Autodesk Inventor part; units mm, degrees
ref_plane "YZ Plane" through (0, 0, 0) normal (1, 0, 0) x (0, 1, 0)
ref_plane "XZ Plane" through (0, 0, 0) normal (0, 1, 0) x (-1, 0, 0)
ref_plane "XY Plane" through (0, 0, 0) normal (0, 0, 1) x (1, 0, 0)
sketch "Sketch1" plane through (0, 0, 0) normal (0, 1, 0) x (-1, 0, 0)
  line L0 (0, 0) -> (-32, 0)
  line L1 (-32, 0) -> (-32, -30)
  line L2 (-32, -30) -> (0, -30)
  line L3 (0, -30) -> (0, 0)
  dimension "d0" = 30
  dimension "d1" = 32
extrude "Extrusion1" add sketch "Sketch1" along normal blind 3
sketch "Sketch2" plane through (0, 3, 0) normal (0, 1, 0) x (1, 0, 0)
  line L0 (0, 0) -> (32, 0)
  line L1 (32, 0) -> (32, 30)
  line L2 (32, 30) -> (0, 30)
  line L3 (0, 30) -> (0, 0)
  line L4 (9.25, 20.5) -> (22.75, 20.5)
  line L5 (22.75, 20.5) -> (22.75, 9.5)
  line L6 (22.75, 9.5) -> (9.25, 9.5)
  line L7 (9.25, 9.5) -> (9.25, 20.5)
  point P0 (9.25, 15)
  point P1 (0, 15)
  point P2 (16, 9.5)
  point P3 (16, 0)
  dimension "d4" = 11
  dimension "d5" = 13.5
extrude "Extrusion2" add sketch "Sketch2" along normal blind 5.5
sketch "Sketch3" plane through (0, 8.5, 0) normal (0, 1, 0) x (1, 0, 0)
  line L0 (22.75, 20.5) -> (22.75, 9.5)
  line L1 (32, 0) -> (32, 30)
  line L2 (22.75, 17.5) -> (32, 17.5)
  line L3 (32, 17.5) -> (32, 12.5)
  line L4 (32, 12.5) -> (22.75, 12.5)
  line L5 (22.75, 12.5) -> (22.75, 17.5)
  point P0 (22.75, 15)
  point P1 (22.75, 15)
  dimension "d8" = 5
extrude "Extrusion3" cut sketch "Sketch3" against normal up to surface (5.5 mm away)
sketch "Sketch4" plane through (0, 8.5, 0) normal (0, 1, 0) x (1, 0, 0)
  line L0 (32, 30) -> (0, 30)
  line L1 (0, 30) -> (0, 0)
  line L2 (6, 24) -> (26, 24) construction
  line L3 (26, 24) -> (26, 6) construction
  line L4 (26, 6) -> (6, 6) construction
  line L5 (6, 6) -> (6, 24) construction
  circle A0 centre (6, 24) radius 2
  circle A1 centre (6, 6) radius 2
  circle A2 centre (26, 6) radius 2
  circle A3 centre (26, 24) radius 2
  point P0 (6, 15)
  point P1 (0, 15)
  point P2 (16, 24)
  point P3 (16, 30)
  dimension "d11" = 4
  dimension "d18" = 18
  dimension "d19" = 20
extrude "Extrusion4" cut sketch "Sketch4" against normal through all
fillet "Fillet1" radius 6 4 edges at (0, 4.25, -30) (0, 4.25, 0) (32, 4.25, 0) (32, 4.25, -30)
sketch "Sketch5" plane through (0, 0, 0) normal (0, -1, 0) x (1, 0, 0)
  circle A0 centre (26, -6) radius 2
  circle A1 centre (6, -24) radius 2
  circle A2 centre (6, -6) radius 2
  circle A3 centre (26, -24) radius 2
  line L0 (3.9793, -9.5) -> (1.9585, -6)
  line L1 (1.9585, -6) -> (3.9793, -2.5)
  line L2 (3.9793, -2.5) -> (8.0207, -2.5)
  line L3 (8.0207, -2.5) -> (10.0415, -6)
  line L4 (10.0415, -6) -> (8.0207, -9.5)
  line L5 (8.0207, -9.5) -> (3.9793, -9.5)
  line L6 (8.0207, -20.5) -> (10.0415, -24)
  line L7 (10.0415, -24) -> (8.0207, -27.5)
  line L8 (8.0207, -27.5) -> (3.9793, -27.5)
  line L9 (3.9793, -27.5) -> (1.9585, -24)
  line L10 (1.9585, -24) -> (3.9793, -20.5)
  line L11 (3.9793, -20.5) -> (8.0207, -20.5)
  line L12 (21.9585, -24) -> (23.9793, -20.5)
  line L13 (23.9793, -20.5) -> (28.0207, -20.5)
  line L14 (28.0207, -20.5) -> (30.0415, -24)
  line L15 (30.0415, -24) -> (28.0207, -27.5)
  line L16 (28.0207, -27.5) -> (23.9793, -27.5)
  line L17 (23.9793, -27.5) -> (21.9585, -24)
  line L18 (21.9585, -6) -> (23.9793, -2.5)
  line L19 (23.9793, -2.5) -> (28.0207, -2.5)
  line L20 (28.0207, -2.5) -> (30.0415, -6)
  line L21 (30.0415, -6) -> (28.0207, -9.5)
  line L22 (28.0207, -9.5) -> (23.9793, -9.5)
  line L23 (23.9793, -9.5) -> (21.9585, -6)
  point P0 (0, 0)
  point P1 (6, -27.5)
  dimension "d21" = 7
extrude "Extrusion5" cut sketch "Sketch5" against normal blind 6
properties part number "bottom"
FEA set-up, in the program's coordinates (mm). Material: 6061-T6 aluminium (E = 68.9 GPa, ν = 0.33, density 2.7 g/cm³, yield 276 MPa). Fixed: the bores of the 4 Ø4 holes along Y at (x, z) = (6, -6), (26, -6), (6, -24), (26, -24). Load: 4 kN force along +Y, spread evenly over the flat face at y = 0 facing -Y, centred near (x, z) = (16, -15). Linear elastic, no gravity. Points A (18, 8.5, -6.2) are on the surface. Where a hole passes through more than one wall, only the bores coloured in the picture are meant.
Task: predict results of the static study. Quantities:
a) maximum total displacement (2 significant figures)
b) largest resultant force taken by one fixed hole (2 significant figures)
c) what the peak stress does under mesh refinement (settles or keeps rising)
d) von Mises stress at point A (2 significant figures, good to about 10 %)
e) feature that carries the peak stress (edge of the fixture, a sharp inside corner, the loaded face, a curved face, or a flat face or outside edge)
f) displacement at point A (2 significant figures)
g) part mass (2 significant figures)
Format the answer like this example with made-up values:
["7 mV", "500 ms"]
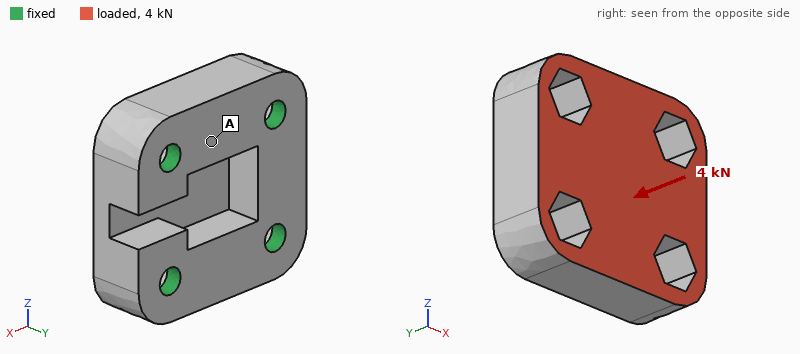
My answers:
["8.7 µm", "1.1 kN", "keeps rising", "12 MPa", "edge of the fixture", "5.2 µm", "15 g"]
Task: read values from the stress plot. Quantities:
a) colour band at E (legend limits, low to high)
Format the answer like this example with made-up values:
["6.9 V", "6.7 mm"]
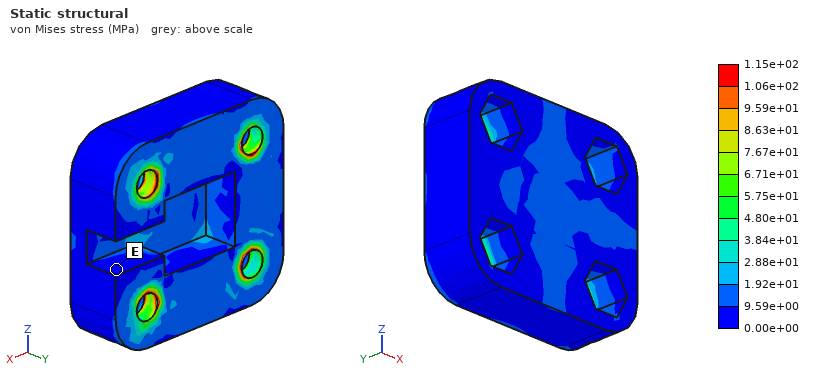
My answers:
["0.00e+00 to 9.59e+00 MPa"]
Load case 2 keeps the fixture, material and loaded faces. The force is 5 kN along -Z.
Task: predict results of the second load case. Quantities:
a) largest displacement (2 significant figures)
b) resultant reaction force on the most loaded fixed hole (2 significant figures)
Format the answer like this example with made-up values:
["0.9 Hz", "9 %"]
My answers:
["20 µm", "1.7 kN"]
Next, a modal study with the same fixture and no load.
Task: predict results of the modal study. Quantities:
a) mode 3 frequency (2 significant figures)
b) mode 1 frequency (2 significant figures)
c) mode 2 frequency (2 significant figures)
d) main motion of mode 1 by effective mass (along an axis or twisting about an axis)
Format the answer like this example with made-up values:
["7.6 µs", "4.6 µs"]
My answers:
["39 kHz", "33 kHz", "38 kHz", "along Z"]
